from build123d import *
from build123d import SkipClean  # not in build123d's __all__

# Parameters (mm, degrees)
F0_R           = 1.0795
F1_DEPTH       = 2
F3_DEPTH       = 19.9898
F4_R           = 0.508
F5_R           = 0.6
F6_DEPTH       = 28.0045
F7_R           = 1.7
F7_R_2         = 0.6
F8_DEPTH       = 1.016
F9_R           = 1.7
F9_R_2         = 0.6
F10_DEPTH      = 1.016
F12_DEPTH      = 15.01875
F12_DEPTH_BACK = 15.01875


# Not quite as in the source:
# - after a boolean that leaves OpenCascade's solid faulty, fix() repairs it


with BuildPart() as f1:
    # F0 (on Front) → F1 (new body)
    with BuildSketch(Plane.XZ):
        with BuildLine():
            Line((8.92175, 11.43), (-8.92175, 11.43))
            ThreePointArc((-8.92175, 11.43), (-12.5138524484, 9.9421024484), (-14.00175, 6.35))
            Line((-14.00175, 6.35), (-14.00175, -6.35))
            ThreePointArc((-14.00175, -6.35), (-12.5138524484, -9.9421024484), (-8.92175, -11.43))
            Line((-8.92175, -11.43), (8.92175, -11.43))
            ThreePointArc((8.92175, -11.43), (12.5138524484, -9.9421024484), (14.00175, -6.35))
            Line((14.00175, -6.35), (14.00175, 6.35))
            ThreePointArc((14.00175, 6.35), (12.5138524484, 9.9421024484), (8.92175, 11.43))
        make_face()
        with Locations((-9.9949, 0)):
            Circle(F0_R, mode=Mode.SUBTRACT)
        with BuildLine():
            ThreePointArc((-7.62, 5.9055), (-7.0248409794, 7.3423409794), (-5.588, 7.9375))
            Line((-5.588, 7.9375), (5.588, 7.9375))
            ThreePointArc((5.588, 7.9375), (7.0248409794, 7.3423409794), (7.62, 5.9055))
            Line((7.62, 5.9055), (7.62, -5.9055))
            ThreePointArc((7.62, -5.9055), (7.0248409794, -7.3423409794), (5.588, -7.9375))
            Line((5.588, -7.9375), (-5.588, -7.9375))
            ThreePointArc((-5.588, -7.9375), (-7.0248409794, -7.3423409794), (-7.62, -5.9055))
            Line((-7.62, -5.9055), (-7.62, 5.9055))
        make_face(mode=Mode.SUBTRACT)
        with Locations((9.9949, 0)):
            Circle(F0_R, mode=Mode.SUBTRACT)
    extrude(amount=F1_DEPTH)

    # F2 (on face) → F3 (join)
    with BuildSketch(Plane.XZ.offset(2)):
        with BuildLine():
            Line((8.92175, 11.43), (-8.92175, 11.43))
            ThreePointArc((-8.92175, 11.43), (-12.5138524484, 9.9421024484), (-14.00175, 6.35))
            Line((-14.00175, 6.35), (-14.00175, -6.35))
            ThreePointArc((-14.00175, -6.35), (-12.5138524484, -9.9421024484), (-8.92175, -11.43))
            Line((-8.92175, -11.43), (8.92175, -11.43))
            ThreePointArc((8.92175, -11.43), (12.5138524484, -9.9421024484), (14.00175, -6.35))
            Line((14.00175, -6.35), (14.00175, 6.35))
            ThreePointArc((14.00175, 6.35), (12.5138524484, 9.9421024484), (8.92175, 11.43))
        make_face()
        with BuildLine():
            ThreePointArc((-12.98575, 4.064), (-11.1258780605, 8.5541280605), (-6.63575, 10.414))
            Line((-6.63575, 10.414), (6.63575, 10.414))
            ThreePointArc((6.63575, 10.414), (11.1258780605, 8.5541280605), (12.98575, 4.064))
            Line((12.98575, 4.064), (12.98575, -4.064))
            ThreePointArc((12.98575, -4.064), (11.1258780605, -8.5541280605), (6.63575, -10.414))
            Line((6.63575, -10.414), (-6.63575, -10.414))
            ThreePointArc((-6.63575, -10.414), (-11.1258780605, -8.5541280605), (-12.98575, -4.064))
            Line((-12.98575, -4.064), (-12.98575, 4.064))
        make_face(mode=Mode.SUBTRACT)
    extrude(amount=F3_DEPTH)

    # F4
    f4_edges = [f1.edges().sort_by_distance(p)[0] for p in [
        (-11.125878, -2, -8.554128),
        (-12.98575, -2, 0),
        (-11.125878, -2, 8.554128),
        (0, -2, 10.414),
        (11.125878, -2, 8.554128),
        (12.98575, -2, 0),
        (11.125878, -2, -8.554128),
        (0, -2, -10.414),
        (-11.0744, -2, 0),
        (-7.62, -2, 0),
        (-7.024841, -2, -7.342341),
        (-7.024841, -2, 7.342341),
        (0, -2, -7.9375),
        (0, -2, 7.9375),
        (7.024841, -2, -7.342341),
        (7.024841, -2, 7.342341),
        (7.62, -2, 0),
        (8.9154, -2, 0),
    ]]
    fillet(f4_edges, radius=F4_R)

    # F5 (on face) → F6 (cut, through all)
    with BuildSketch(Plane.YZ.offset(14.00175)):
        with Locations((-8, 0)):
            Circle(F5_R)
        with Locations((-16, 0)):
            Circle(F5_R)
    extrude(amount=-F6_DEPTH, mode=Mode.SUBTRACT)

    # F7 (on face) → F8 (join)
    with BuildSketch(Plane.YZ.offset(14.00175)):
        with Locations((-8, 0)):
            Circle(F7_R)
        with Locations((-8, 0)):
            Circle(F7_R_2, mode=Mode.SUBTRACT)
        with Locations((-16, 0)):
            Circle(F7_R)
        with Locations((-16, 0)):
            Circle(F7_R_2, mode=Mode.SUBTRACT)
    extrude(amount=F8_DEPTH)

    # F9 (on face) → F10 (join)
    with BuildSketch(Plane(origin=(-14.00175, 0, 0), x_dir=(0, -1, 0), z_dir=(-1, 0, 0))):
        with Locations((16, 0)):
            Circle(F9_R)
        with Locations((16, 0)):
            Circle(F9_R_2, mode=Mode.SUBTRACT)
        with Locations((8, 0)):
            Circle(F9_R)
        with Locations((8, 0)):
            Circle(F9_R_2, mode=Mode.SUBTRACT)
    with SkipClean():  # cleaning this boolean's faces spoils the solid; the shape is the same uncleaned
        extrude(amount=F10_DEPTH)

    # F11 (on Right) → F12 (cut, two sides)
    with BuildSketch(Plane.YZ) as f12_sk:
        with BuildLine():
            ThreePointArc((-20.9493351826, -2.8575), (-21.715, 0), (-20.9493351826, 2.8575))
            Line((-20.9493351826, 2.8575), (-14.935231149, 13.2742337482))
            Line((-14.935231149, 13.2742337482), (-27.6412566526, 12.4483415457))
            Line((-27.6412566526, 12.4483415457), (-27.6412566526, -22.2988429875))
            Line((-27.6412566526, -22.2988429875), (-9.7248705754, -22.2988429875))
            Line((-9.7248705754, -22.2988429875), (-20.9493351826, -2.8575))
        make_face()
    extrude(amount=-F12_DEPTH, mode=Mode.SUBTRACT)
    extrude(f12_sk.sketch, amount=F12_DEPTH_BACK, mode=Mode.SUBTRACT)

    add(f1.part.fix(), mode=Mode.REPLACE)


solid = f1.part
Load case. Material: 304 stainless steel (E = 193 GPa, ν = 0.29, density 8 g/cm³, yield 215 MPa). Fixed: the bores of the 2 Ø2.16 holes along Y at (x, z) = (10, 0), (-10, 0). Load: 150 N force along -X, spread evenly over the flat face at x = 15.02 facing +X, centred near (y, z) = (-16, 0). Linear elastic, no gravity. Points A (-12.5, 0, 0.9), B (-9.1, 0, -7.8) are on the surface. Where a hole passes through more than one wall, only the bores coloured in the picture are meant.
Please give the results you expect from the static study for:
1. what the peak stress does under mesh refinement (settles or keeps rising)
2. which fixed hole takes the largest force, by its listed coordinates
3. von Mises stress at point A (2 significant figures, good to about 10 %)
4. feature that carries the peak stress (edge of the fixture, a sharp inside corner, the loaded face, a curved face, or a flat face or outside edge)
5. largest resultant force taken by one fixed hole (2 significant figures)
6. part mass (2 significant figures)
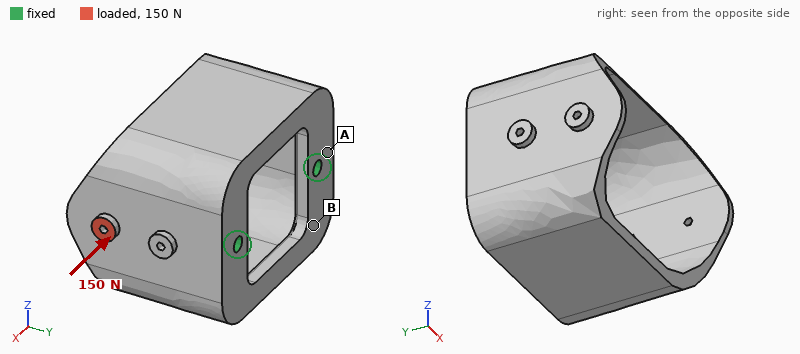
keeps rising
(10, 0)
18 MPa
a sharp inside corner
150 N
20 g
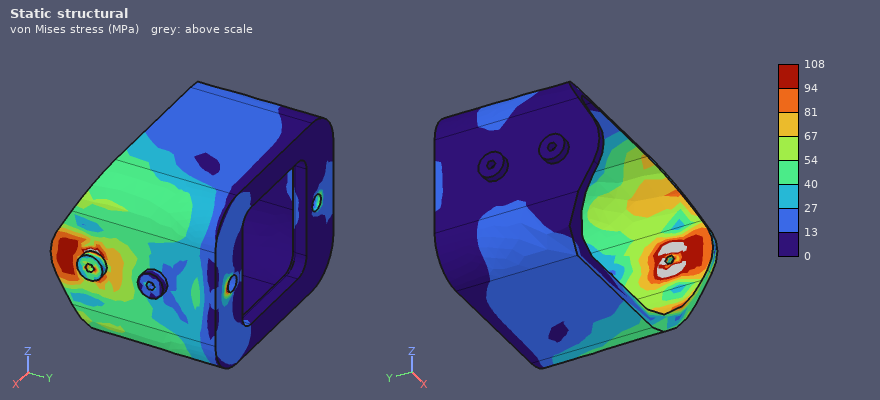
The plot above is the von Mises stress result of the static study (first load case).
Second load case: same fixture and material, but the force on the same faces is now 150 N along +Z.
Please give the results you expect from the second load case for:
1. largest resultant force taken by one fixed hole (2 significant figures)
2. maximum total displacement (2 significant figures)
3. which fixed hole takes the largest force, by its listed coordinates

160 N
52 µm
(10, 0)
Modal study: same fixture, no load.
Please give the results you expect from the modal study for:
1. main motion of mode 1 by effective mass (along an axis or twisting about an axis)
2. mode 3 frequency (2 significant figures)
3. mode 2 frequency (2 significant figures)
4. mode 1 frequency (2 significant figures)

along Z
7700 Hz
5100 Hz
3400 Hz
